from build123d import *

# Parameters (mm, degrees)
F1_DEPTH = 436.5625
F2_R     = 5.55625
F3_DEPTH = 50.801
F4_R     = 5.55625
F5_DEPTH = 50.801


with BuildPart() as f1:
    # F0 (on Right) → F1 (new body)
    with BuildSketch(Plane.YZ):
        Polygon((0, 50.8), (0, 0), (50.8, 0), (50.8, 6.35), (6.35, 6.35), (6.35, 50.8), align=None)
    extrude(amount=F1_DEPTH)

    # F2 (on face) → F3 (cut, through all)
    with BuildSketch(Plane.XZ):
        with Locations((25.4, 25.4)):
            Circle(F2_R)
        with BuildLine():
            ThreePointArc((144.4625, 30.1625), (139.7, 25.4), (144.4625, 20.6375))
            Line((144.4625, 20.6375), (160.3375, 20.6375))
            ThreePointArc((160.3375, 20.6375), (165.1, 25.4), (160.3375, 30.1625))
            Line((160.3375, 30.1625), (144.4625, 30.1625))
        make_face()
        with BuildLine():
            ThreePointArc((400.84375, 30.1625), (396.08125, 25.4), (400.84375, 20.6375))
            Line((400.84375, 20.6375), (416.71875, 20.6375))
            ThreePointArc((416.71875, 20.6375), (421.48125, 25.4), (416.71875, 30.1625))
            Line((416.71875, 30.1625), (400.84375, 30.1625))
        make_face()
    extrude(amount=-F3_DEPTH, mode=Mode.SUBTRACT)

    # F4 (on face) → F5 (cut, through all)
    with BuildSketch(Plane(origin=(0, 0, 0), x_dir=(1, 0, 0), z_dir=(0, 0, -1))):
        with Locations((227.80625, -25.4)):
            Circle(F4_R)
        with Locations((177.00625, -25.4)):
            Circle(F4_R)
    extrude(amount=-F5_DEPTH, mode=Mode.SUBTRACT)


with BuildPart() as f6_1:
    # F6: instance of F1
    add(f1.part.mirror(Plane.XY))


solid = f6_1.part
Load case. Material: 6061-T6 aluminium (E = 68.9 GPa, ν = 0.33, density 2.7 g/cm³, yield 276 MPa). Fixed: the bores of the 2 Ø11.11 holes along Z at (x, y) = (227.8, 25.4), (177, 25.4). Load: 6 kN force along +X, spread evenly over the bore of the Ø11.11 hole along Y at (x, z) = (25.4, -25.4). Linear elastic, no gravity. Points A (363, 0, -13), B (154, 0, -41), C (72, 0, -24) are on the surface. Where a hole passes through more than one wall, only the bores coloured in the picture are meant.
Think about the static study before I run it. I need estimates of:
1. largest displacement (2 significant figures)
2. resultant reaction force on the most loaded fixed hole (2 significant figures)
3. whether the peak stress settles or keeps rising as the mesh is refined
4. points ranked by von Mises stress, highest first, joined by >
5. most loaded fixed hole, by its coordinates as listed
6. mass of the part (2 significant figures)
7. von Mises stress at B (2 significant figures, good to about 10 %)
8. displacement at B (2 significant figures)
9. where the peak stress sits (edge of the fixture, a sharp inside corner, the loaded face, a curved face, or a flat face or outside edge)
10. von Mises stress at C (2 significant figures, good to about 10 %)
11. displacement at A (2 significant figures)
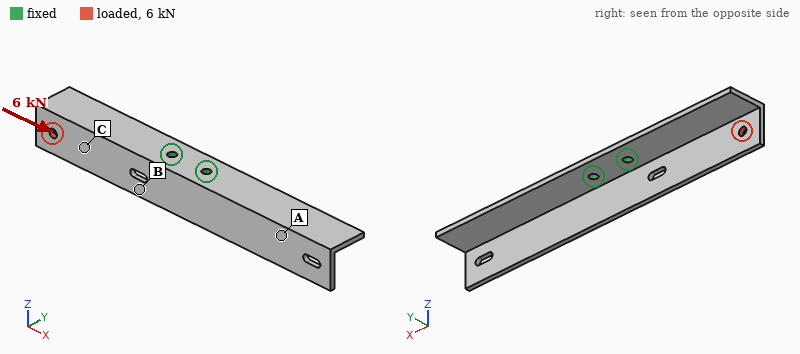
0.54 mm
4.5 kN
keeps rising
B > C > A
(177, 25.4)
700 g
33 MPa
0.17 mm
edge of the fixture
18 MPa
0.35 mm
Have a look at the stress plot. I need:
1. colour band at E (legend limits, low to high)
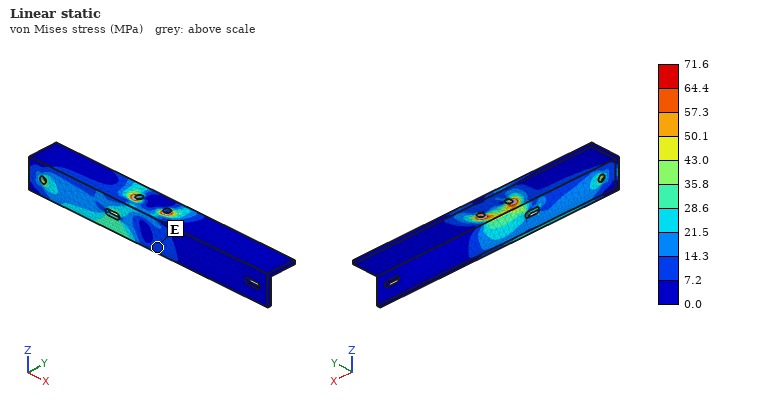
7.2 to 14.3 MPa
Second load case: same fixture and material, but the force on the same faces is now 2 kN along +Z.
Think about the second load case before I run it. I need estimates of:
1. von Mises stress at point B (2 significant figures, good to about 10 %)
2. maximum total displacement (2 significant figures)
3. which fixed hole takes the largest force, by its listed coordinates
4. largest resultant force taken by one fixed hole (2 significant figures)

76 MPa
2.0 mm
(177, 25.4)
6.8 kN
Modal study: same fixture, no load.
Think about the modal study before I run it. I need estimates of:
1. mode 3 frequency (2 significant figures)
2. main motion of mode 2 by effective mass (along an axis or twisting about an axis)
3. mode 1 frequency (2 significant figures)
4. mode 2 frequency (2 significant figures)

570 Hz
along Y
350 Hz
490 Hz
